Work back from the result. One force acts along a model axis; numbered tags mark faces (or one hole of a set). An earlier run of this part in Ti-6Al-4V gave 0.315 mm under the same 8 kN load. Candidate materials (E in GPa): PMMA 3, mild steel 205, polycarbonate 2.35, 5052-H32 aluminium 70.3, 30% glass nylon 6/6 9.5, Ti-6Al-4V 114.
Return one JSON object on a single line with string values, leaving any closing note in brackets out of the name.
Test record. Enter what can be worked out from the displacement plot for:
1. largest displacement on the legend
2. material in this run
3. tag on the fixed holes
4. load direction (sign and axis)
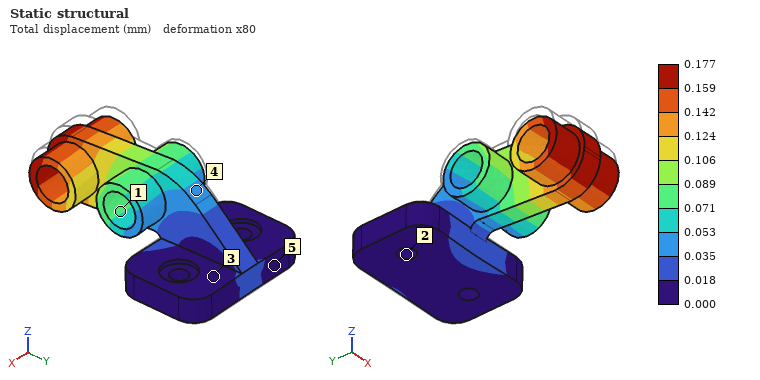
{"largest displacement on the legend": "0.177 mm", "material in this run": "mild steel", "tag on the fixed holes": "2", "load direction": "-Z"}
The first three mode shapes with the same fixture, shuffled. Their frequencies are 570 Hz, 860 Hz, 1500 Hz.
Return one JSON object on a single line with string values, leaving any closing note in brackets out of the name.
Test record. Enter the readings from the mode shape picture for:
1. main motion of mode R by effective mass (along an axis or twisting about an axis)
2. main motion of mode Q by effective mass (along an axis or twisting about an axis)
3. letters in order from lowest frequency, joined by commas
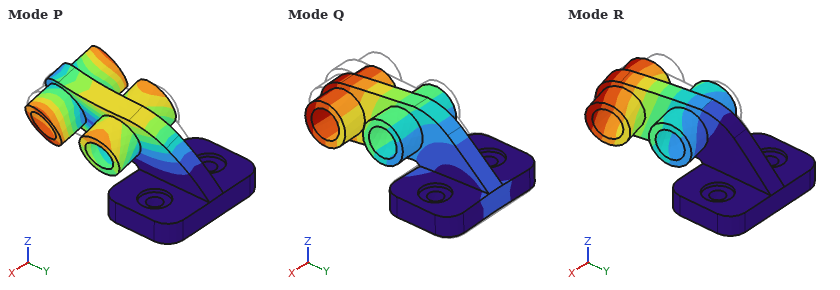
{"main motion of mode R by effective mass": "along X", "main motion of mode Q by effective mass": "along Z", "letters in order from lowest frequency, joined by commas": "R, Q, P"}
